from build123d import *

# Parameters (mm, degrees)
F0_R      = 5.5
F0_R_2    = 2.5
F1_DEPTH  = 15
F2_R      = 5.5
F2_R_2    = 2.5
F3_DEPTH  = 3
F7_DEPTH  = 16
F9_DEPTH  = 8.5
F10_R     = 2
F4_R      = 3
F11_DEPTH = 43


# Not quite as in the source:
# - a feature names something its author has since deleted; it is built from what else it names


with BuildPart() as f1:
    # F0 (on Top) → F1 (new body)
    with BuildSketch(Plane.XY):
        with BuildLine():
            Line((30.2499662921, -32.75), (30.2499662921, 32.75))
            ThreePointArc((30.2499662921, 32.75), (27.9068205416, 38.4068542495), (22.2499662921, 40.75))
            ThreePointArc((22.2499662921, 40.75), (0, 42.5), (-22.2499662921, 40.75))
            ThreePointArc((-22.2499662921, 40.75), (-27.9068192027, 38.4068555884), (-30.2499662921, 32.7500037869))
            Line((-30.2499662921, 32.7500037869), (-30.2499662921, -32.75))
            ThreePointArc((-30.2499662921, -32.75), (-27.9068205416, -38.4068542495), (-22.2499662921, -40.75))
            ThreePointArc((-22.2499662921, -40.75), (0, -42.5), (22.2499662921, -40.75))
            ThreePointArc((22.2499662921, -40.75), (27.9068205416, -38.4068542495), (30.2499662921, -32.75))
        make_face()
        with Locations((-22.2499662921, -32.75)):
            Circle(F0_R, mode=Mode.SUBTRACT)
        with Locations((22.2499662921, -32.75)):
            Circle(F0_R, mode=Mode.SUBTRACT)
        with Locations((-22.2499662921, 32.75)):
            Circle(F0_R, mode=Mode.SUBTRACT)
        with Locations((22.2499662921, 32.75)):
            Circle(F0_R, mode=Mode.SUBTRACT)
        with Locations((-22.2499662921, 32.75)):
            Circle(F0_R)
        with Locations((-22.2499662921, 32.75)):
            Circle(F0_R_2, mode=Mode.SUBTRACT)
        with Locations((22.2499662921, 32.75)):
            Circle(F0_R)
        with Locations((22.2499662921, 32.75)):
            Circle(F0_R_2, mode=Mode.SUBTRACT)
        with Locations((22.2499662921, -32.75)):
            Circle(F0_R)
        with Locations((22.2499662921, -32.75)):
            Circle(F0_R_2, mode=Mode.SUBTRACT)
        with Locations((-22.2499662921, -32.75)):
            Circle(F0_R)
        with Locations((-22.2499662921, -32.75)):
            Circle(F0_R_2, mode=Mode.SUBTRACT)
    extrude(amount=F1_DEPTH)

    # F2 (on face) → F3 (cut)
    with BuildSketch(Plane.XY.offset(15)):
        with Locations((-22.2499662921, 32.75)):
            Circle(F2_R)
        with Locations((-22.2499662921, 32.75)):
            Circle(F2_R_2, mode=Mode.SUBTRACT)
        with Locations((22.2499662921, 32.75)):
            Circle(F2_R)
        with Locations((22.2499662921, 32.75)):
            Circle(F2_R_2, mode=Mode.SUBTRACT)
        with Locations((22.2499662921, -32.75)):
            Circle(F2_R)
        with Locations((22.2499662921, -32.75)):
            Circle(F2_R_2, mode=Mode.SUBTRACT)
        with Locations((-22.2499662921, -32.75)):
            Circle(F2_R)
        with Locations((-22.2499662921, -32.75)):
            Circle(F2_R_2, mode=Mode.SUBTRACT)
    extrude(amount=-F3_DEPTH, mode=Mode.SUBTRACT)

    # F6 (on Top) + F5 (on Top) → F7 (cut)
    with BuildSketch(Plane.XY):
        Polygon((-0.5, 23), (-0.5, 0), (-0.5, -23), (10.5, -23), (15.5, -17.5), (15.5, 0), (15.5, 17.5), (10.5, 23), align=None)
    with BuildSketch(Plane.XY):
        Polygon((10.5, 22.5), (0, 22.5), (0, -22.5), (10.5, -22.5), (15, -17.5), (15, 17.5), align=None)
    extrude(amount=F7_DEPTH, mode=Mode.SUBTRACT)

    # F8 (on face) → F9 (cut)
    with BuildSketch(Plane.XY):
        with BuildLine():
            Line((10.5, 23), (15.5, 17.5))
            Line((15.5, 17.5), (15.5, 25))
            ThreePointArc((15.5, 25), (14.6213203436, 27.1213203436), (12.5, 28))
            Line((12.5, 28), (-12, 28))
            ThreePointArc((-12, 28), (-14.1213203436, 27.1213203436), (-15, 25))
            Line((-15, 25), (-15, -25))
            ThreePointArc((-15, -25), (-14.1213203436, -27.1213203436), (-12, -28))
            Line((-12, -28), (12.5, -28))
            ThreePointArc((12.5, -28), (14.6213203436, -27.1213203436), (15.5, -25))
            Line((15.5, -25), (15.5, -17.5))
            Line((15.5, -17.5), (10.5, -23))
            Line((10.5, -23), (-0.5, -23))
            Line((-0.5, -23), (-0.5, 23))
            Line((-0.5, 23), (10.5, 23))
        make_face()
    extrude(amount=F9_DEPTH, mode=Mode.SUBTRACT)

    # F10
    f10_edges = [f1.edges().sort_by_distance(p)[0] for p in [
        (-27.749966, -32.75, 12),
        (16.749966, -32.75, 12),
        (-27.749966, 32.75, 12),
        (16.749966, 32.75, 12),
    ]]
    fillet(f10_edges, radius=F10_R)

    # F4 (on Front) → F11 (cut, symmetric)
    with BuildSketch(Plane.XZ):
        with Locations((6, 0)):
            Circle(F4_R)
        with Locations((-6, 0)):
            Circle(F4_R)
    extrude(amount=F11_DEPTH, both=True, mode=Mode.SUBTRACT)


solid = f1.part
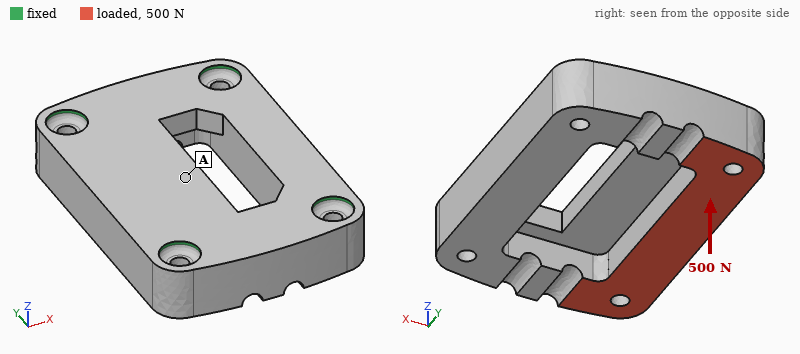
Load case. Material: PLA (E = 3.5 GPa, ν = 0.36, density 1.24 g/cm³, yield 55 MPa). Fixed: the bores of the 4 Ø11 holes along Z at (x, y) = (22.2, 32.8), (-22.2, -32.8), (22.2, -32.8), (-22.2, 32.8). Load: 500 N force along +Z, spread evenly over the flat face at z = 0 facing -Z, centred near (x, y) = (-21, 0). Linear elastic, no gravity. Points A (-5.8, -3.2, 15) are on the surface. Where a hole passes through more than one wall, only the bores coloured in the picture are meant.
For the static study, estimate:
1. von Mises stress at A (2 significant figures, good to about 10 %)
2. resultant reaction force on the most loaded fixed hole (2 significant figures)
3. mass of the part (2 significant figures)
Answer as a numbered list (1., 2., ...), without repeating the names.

1. 0.85 MPa
2. 270 N
3. 66 g
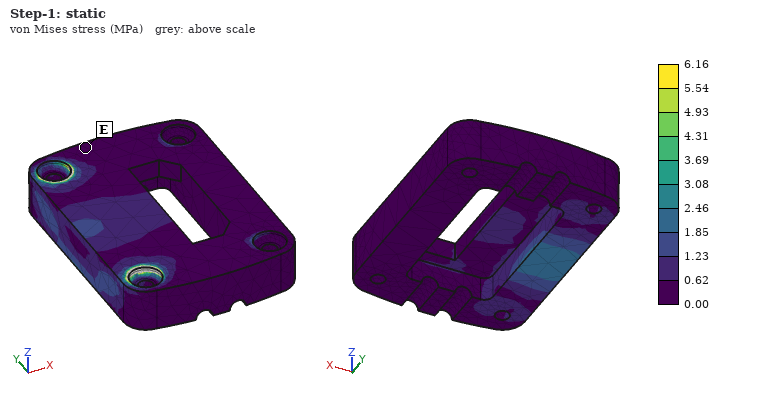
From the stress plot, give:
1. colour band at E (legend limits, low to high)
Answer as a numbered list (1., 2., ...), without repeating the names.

1. 0.00 to 0.62 MPa
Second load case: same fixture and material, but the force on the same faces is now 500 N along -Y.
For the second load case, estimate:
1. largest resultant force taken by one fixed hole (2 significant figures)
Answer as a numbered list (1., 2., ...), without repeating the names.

1. 240 N
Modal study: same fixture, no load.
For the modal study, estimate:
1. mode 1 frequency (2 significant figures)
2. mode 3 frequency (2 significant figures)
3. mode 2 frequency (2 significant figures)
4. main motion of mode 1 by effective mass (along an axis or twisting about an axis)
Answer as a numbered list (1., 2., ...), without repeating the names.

1. 3400 Hz
2. 4300 Hz
3. 4100 Hz
4. along Z
